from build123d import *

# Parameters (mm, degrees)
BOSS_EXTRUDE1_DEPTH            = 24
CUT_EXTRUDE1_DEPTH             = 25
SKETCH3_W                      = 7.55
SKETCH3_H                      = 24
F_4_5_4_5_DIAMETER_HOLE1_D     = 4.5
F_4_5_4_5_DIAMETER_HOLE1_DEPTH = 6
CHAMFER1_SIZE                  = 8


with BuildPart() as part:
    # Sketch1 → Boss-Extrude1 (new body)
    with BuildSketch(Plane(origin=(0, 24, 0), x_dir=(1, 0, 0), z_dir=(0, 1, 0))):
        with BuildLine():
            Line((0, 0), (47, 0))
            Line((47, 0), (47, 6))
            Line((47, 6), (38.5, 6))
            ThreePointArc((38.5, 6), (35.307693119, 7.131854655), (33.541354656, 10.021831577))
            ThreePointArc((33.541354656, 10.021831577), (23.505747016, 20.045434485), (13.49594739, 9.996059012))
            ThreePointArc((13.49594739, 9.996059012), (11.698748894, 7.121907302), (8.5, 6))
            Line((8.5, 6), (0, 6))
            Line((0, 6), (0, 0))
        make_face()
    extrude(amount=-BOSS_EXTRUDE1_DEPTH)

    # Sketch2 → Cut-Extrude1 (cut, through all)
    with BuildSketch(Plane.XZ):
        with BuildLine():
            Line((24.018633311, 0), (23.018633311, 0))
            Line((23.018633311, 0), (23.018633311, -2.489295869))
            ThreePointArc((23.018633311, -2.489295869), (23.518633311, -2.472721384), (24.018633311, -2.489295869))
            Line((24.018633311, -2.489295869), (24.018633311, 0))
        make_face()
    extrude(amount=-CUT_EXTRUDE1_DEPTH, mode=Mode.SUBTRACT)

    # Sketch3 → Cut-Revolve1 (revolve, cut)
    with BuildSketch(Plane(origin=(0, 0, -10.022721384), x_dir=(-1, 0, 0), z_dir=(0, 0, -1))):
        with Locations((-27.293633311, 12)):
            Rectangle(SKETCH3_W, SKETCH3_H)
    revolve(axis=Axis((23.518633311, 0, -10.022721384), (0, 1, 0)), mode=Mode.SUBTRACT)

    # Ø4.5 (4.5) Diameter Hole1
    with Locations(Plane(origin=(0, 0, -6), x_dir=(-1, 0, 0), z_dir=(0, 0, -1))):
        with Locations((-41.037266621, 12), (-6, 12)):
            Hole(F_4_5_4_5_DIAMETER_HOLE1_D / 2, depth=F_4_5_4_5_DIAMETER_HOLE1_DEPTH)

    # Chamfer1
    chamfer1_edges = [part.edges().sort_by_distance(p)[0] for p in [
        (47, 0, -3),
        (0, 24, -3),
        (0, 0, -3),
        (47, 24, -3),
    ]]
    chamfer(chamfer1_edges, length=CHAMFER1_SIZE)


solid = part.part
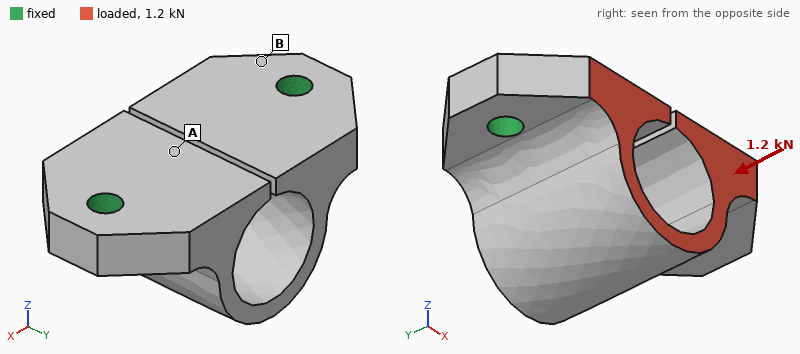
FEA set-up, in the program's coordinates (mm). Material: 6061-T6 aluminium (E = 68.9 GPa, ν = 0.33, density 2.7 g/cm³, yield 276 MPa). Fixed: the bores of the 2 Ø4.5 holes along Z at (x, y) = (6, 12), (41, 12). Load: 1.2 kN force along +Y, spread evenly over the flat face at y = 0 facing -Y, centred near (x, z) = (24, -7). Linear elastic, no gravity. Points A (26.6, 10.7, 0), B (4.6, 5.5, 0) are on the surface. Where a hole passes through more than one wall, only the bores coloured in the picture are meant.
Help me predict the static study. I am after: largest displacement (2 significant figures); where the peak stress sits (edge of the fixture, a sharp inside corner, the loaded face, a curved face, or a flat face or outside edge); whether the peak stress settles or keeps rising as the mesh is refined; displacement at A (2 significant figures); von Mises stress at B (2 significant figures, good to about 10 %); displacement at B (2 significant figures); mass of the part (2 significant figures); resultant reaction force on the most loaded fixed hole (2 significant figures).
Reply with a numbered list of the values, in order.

1. 20 µm
2. edge of the fixture
3. keeps rising
4. 7.2 µm
5. 13 MPa
6. 3.6 µm
7. 20 g
8. 600 N
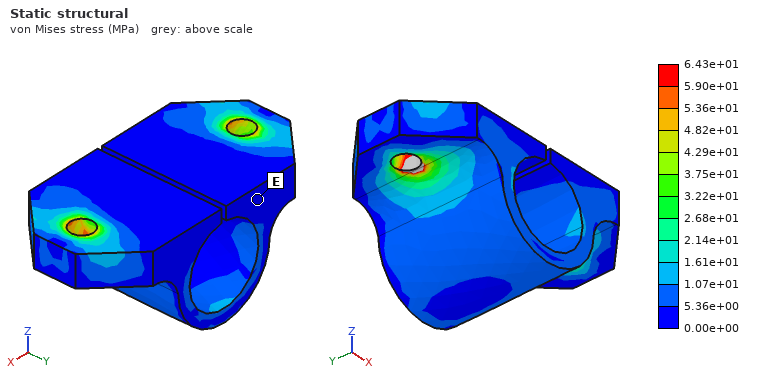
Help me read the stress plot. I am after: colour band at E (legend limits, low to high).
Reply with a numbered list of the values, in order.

1. 0.00e+00 to 5.36e+00 MPa
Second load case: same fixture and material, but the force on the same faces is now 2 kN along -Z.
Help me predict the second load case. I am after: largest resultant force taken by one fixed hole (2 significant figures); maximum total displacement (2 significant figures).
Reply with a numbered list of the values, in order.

1. 1.0 kN
2. 59 µm
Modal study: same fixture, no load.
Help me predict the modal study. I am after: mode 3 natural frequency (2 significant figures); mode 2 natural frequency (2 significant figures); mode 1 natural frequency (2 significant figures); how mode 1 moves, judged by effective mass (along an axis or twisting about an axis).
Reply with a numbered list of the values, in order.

1. 16 kHz
2. 14 kHz
3. 11 kHz
4. along Y
